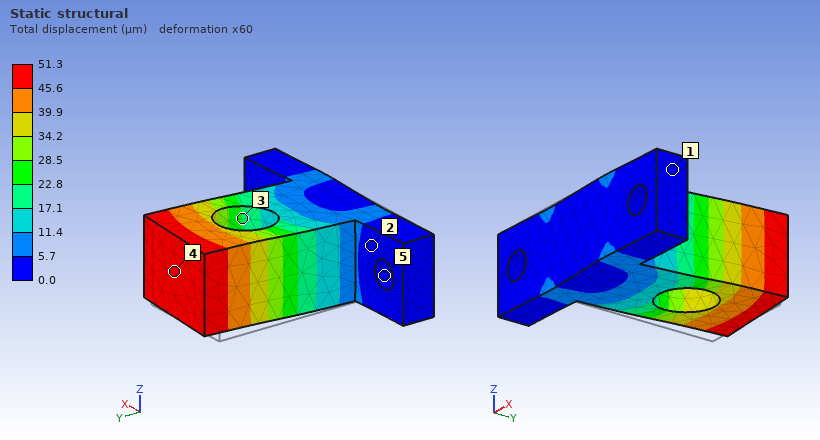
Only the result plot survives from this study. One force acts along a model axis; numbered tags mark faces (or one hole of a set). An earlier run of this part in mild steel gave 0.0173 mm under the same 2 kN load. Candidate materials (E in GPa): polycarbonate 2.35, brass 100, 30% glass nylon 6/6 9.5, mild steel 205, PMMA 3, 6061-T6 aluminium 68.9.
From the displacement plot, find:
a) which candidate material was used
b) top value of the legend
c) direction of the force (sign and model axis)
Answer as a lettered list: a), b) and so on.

a) 6061-T6 aluminium
b) 51.3 µm
c) +X
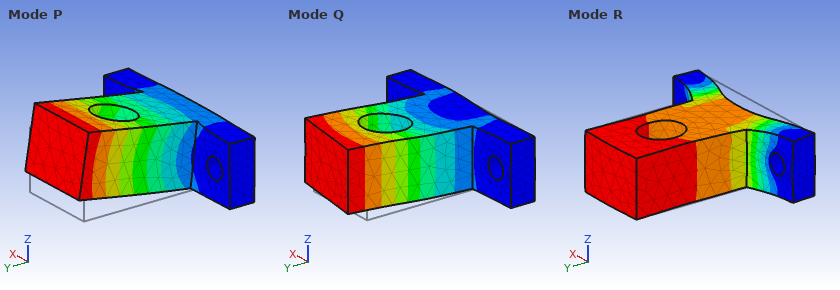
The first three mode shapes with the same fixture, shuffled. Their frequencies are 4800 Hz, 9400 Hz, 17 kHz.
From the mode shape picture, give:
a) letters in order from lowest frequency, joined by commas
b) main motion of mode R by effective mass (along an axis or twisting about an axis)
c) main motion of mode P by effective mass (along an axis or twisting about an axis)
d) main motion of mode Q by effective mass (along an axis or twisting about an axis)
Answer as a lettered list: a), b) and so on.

a) P, Q, R
b) along Y
c) along Z
d) along X
